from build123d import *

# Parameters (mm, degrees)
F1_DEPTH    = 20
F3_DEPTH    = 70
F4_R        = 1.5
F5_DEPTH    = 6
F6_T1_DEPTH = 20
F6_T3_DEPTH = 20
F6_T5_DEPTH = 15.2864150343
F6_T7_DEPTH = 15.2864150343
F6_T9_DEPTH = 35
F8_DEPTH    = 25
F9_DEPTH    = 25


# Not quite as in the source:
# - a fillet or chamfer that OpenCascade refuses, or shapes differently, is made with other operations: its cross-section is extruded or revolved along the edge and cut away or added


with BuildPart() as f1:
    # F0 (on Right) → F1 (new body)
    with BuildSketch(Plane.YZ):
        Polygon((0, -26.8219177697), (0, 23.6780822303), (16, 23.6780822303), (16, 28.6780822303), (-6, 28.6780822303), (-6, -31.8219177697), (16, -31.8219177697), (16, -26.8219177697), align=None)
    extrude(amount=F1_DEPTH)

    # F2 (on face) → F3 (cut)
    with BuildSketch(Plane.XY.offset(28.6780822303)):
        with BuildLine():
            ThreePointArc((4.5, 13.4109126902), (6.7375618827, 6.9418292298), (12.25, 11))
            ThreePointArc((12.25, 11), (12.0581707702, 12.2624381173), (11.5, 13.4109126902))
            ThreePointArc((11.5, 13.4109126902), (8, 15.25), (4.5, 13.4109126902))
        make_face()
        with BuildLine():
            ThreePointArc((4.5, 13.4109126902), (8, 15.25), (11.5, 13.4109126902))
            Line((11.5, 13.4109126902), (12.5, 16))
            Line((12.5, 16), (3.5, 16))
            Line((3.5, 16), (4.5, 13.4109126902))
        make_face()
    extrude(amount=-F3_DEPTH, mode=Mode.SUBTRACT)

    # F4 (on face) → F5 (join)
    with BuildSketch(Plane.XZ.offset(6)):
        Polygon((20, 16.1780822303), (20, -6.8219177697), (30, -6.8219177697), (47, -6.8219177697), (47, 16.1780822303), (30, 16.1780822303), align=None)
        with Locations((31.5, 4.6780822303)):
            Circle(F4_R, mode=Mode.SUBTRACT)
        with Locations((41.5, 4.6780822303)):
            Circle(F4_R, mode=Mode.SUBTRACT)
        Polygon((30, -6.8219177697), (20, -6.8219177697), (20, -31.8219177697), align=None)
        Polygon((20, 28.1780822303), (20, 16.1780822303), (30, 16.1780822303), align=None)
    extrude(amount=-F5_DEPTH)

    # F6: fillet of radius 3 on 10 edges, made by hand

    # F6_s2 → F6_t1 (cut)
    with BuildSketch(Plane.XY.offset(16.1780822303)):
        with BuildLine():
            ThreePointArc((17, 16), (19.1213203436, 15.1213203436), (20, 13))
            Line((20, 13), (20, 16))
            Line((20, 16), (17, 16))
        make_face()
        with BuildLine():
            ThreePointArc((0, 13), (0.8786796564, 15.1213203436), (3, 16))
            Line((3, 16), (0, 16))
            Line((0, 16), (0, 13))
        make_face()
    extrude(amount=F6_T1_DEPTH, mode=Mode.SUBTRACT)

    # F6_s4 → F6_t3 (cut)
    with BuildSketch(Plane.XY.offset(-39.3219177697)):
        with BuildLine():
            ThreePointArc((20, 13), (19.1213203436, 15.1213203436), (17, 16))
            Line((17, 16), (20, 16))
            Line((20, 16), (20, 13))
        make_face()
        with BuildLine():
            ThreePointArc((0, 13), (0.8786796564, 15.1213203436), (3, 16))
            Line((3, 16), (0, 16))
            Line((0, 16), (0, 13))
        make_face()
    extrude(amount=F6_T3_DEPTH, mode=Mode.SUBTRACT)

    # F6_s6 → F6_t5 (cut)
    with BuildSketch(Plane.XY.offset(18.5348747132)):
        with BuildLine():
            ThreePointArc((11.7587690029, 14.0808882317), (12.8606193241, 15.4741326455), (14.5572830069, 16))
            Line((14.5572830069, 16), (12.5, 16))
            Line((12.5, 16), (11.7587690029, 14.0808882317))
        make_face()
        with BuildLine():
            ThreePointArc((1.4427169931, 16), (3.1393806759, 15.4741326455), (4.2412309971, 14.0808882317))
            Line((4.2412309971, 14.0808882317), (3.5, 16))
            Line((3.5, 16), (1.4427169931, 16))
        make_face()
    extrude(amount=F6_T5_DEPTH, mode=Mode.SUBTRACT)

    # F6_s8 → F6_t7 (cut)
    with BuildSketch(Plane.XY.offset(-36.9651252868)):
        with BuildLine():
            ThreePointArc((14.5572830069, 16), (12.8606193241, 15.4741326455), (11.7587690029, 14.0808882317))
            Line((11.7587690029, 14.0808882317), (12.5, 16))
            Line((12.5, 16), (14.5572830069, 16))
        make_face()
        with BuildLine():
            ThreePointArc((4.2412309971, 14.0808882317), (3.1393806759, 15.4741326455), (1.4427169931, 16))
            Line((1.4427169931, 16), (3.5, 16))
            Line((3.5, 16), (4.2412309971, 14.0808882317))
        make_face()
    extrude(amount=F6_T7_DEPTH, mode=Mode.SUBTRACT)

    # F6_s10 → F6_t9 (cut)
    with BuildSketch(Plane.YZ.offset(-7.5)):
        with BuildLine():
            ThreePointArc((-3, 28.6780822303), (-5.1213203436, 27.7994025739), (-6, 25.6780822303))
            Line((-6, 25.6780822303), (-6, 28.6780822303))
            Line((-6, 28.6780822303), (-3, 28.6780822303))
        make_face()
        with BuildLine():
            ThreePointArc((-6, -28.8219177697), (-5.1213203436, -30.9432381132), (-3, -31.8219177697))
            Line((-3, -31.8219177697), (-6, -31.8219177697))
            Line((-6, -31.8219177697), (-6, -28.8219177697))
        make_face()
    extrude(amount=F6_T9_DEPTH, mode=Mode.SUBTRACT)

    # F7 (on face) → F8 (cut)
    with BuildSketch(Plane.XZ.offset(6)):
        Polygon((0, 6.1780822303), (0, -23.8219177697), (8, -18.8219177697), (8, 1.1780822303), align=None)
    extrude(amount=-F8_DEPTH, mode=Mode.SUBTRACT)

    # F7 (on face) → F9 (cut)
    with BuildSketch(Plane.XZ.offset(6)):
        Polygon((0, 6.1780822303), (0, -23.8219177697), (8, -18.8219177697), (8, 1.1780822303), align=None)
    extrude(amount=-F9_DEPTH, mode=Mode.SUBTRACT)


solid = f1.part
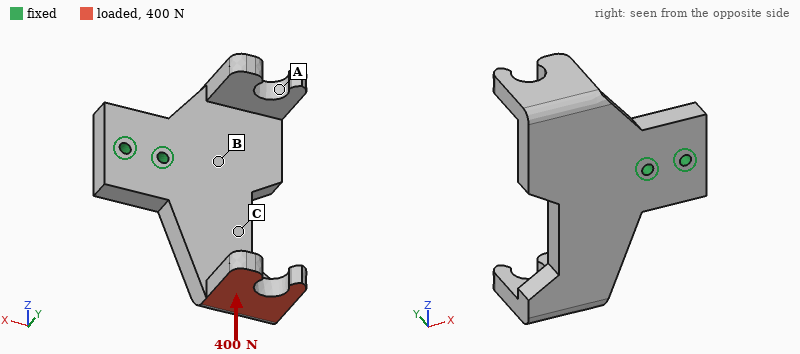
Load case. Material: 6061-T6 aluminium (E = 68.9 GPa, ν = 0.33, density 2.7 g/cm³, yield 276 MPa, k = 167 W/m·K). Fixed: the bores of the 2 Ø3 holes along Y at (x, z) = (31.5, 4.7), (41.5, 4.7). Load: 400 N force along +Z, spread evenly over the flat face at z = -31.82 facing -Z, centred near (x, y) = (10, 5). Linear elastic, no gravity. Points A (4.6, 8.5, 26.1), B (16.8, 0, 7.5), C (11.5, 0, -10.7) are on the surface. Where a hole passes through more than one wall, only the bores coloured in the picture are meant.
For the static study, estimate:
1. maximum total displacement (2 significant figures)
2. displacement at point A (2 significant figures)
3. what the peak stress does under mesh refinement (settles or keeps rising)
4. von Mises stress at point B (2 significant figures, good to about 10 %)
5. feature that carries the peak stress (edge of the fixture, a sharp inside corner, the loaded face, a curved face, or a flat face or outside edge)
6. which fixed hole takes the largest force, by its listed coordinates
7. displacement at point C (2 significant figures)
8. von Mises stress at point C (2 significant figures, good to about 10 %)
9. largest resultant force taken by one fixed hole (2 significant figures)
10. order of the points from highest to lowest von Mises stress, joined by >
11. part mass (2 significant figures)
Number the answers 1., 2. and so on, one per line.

1. 0.17 mm
2. 0.033 mm
3. keeps rising
4. 13 MPa
5. edge of the fixture
6. (31.5, 4.7)
7. 0.031 mm
8. 35 MPa
9. 1.0 kN
10. C > B > A
11. 36 g
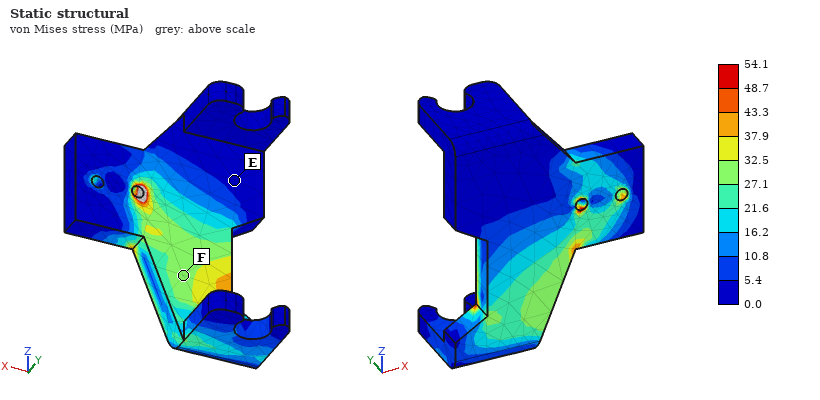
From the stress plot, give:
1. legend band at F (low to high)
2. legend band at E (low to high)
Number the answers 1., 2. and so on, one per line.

1. 27.1 to 32.5 MPa
2. 0.0 to 5.4 MPa
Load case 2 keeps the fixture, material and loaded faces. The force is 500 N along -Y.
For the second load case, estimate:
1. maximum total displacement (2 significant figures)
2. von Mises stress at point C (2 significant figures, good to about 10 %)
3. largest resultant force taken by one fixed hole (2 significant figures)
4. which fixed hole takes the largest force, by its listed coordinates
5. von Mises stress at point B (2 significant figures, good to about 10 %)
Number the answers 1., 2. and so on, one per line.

1. 0.67 mm
2. 89 MPa
3. 890 N
4. (31.5, 4.7)
5. 56 MPa
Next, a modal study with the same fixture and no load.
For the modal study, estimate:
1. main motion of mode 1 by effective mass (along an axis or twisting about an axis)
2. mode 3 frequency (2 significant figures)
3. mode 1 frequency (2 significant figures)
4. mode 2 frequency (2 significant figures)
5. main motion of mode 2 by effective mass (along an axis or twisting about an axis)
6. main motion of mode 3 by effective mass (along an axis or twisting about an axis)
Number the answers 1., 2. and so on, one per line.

1. along Y
2. 3900 Hz
3. 1900 Hz
4. 2800 Hz
5. along Y
6. along Z
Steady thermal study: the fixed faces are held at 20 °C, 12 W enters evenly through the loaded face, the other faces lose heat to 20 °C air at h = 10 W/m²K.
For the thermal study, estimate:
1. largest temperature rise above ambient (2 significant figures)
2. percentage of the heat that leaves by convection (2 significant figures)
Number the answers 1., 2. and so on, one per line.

1. 30 K
2. 4.4 %
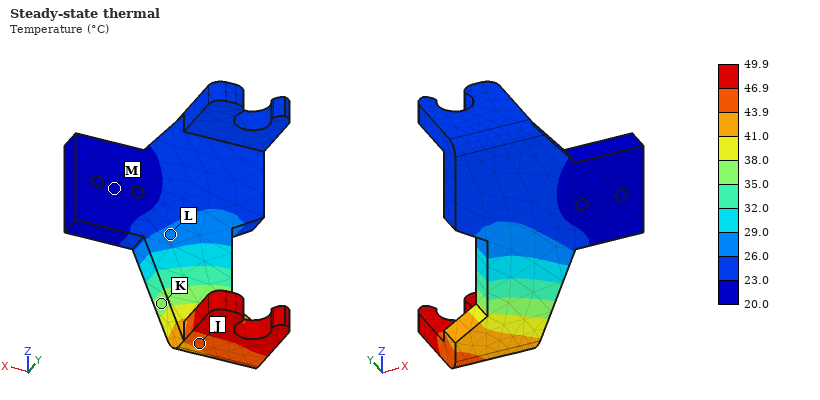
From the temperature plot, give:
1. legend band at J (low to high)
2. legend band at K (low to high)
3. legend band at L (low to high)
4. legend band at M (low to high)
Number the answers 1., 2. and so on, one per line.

1. 43.9 to 46.9 °C
2. 35.0 to 38.0 °C
3. 26.0 to 29.0 °C
4. 20.0 to 23.0 °C
